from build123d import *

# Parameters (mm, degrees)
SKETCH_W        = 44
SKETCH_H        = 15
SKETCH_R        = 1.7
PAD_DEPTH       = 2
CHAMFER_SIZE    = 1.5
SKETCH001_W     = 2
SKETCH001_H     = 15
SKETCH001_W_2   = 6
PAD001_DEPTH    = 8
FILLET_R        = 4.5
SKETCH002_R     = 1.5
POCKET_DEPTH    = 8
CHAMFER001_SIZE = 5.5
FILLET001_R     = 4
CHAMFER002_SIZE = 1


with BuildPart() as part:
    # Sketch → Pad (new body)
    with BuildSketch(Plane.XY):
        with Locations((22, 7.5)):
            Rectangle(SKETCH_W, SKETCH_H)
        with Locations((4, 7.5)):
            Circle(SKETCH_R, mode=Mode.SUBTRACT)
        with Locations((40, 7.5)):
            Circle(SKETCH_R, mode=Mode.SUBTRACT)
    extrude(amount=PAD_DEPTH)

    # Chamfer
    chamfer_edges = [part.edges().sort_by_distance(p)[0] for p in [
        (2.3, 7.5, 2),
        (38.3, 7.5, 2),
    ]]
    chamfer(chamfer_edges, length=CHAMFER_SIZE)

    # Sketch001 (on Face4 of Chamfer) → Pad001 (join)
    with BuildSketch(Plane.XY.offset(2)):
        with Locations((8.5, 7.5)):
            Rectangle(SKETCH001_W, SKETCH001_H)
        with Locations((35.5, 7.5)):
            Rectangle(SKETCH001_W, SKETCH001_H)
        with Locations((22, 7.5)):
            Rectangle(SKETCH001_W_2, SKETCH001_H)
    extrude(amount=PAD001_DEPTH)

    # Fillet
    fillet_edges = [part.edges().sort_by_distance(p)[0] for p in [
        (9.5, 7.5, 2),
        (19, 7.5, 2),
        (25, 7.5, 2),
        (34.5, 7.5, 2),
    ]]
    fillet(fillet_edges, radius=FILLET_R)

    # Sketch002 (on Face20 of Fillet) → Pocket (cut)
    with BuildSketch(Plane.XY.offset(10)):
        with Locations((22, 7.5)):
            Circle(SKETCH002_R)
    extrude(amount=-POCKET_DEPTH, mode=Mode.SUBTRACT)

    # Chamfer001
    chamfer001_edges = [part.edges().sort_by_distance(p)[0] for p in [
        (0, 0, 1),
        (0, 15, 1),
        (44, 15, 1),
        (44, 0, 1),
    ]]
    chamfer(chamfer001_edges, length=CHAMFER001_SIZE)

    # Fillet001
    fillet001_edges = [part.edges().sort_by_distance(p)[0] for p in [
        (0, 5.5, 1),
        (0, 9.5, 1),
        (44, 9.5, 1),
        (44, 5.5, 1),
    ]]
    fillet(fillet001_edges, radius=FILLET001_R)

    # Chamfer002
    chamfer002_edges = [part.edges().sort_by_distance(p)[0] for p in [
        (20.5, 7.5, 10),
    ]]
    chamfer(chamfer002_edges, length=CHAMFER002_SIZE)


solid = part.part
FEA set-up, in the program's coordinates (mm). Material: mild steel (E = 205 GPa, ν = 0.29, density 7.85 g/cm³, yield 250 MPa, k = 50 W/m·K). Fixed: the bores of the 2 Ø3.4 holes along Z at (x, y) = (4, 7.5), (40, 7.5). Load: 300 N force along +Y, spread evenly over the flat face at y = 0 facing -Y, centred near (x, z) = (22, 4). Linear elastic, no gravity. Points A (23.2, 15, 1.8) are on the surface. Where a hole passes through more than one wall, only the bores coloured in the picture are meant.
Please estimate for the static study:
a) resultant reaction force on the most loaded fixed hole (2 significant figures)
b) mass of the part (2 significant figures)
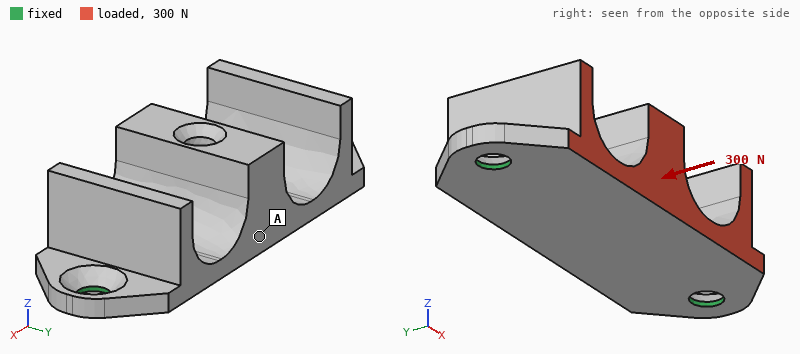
150 N
20 g
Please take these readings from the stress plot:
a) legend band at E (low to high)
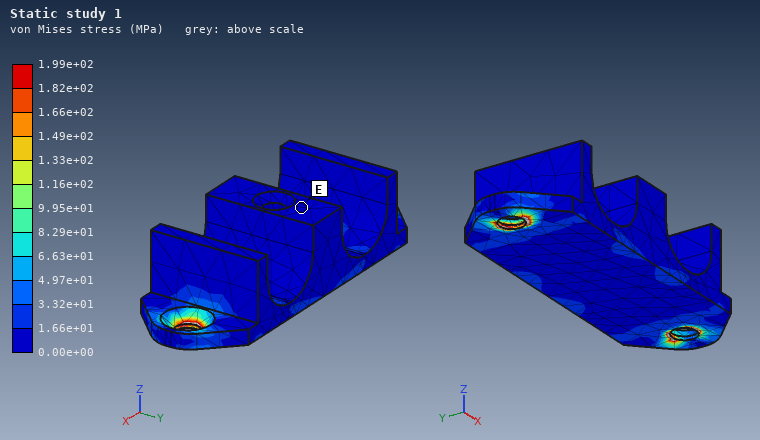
0.00e+00 to 1.66e+01 MPa
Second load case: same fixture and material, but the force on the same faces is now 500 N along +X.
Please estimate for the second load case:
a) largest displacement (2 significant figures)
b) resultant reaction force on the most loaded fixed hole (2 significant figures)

3.4 µm
270 N
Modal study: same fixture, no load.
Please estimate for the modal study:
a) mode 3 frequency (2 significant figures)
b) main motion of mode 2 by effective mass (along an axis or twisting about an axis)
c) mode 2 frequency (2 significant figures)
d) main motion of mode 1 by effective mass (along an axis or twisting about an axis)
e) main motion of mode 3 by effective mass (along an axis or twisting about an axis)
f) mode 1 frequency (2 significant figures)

12 kHz
along Z
5600 Hz
along Y
twisting about Y
4700 Hz
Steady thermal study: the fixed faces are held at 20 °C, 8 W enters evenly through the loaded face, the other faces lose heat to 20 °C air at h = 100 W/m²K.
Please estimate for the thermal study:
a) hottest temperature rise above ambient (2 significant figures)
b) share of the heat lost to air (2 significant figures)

27 K
39 %
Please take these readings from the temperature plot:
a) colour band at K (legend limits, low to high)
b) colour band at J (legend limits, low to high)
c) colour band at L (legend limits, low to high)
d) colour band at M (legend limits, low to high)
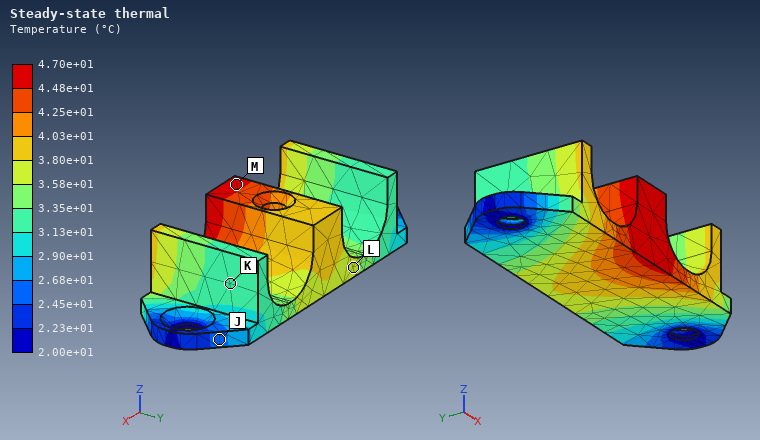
3.13e+01 to 3.35e+01 °C
2.45e+01 to 2.68e+01 °C
3.58e+01 to 3.80e+01 °C
4.48e+01 to 4.70e+01 °C
